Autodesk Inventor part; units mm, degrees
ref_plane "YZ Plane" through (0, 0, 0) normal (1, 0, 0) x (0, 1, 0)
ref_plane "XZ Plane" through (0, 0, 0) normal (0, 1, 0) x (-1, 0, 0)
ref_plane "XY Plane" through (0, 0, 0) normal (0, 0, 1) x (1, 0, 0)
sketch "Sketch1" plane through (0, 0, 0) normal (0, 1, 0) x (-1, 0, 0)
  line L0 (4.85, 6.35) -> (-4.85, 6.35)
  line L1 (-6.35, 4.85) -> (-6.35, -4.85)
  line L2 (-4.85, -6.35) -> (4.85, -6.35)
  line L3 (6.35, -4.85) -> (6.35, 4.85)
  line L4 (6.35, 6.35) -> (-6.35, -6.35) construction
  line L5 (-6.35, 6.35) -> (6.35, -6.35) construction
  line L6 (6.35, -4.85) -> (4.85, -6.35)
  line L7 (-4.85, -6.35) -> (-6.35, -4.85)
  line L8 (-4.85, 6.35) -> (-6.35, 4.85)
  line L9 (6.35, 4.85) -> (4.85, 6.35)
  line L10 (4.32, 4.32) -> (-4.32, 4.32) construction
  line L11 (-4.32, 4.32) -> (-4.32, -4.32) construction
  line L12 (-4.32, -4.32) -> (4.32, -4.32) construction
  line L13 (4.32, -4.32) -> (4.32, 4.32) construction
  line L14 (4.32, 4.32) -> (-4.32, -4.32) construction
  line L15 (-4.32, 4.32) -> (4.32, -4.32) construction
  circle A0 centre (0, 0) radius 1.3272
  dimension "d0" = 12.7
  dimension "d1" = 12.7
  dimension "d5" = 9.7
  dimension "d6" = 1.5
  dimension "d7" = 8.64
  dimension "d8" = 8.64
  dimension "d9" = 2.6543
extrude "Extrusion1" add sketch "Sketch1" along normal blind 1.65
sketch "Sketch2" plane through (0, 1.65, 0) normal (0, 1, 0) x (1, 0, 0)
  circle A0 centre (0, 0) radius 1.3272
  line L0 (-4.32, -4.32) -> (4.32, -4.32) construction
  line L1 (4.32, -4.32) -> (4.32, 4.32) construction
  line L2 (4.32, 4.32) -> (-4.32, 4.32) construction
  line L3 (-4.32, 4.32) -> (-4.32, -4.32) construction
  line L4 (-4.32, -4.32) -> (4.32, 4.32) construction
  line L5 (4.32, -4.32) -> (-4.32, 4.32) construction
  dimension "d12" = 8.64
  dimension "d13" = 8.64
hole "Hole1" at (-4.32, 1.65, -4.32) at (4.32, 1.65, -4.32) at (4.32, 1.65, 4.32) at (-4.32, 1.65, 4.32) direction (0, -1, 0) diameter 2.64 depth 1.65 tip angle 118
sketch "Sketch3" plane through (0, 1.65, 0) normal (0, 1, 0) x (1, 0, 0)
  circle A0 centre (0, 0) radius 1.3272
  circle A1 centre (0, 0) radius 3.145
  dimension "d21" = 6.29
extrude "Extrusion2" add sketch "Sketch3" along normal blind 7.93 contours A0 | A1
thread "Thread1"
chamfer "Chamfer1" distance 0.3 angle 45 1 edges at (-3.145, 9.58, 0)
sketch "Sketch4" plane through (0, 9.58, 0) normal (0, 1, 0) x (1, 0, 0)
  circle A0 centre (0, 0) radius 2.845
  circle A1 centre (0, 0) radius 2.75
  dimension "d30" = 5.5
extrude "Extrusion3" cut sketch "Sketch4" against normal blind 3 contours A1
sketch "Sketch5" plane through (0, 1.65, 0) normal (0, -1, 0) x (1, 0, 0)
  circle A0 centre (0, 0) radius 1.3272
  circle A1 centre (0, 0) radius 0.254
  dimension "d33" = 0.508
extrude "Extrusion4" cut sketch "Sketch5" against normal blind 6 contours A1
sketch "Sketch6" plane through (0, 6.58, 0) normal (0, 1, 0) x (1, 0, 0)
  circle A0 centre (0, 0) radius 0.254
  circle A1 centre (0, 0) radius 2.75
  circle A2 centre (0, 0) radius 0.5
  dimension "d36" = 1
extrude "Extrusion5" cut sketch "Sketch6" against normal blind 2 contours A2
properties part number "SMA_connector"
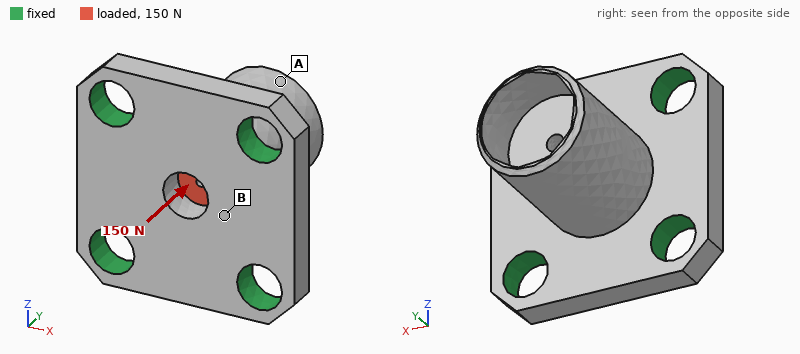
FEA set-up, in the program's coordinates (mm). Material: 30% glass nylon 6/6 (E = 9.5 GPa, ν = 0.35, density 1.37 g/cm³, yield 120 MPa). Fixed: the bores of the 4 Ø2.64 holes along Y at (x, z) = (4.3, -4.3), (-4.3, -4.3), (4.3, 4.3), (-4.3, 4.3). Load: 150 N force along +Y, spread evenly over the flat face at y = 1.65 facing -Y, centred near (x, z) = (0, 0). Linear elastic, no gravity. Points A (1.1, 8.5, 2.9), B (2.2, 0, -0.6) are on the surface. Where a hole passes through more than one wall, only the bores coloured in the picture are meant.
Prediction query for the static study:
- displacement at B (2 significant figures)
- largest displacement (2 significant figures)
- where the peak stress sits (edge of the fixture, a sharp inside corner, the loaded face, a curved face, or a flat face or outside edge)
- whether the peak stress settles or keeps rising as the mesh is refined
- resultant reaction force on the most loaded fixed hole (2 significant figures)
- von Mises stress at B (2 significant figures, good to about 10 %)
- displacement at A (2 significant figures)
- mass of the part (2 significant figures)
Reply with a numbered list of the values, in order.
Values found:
1. 8.5 µm
2. 14 µm
3. edge of the fixture
4. keeps rising
5. 42 N
6. 9.5 MPa
7. 8.7 µm
8. 0.53 g
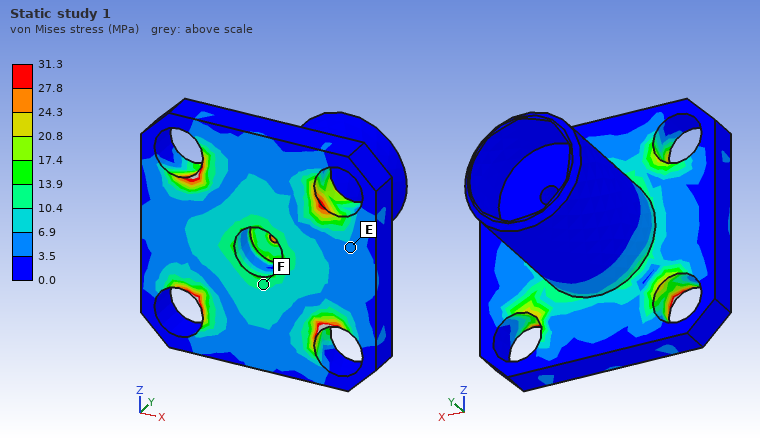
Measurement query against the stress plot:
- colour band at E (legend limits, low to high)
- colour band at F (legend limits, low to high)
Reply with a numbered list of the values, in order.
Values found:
1. 3.5 to 6.9 MPa
2. 10.4 to 13.9 MPa
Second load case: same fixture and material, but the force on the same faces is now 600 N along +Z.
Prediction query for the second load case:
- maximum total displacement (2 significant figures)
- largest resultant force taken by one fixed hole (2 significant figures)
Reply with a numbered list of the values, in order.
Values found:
1. 42 µm
2. 170 N
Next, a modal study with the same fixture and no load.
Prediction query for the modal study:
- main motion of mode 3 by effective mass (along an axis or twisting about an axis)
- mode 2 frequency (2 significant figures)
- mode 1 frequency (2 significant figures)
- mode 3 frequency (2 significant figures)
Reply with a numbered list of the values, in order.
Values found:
1. along Y
2. 25 kHz
3. 25 kHz
4. 37 kHz
